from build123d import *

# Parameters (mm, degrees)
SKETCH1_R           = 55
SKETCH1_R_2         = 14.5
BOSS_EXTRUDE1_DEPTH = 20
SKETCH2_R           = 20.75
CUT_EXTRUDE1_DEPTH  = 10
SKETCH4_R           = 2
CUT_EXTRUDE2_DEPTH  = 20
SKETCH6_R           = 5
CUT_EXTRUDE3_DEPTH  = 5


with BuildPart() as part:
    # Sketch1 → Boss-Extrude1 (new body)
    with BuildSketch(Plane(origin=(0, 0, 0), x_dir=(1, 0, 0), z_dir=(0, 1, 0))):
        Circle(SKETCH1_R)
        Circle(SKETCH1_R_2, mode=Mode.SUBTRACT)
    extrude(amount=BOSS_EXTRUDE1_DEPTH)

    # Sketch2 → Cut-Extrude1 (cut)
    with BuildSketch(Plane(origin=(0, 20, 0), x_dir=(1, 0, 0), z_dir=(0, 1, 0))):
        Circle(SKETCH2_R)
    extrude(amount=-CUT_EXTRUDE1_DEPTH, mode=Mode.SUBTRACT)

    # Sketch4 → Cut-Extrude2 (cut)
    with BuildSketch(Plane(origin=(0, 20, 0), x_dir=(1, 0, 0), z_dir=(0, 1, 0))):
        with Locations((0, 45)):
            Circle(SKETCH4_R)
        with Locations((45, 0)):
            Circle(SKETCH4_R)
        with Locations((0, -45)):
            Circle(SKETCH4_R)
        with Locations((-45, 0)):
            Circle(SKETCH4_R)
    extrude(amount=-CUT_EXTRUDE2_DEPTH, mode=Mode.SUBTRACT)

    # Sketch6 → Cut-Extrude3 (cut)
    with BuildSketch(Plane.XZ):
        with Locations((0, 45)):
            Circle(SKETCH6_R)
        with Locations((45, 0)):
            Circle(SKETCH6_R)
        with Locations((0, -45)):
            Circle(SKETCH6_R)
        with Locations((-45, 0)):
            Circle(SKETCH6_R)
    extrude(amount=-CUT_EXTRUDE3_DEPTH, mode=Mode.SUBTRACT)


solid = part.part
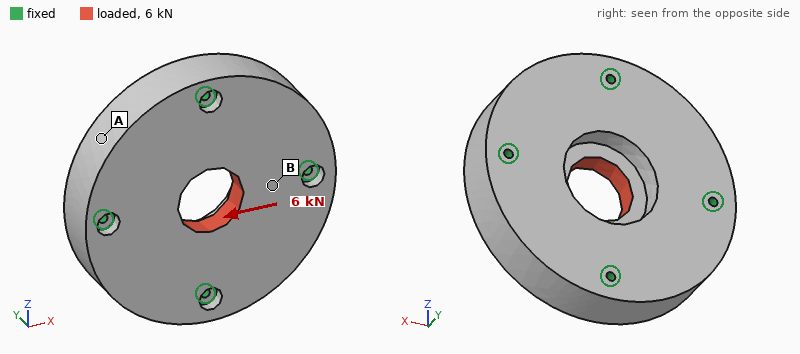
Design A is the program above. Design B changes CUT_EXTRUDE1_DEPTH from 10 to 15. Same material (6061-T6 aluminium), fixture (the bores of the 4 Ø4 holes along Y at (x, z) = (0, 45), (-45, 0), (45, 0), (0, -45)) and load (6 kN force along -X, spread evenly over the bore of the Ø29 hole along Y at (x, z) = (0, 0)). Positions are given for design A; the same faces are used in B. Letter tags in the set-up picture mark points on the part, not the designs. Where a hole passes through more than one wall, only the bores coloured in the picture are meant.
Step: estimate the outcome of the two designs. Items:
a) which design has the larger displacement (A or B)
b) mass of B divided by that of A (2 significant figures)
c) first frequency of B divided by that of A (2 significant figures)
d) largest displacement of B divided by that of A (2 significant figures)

B
0.98
1.00
1.6
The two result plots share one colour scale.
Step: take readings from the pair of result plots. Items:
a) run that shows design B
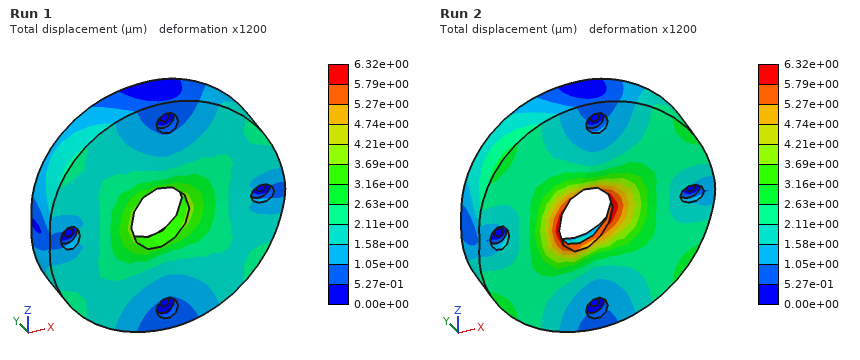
Run 2
